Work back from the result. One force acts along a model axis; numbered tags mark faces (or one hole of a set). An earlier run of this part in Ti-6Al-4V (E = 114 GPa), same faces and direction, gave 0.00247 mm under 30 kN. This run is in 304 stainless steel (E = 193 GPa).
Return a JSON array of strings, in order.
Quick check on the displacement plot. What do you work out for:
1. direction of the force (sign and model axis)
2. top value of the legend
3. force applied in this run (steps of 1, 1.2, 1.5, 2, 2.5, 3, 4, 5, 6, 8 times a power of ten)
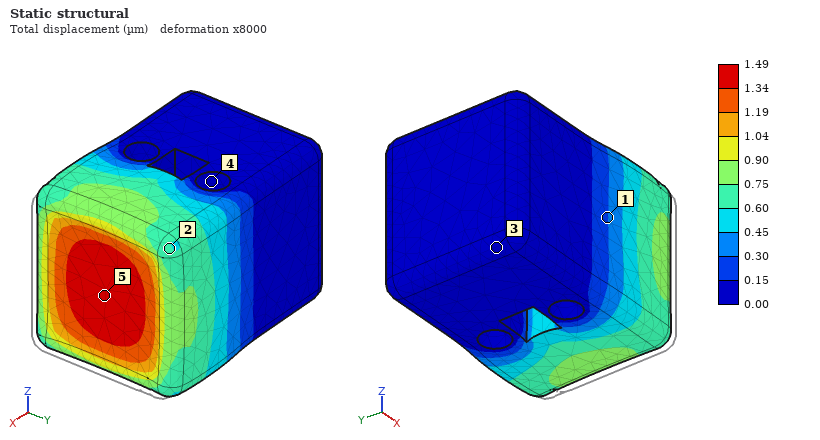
["-X", "1.49 µm", "30 kN"]
